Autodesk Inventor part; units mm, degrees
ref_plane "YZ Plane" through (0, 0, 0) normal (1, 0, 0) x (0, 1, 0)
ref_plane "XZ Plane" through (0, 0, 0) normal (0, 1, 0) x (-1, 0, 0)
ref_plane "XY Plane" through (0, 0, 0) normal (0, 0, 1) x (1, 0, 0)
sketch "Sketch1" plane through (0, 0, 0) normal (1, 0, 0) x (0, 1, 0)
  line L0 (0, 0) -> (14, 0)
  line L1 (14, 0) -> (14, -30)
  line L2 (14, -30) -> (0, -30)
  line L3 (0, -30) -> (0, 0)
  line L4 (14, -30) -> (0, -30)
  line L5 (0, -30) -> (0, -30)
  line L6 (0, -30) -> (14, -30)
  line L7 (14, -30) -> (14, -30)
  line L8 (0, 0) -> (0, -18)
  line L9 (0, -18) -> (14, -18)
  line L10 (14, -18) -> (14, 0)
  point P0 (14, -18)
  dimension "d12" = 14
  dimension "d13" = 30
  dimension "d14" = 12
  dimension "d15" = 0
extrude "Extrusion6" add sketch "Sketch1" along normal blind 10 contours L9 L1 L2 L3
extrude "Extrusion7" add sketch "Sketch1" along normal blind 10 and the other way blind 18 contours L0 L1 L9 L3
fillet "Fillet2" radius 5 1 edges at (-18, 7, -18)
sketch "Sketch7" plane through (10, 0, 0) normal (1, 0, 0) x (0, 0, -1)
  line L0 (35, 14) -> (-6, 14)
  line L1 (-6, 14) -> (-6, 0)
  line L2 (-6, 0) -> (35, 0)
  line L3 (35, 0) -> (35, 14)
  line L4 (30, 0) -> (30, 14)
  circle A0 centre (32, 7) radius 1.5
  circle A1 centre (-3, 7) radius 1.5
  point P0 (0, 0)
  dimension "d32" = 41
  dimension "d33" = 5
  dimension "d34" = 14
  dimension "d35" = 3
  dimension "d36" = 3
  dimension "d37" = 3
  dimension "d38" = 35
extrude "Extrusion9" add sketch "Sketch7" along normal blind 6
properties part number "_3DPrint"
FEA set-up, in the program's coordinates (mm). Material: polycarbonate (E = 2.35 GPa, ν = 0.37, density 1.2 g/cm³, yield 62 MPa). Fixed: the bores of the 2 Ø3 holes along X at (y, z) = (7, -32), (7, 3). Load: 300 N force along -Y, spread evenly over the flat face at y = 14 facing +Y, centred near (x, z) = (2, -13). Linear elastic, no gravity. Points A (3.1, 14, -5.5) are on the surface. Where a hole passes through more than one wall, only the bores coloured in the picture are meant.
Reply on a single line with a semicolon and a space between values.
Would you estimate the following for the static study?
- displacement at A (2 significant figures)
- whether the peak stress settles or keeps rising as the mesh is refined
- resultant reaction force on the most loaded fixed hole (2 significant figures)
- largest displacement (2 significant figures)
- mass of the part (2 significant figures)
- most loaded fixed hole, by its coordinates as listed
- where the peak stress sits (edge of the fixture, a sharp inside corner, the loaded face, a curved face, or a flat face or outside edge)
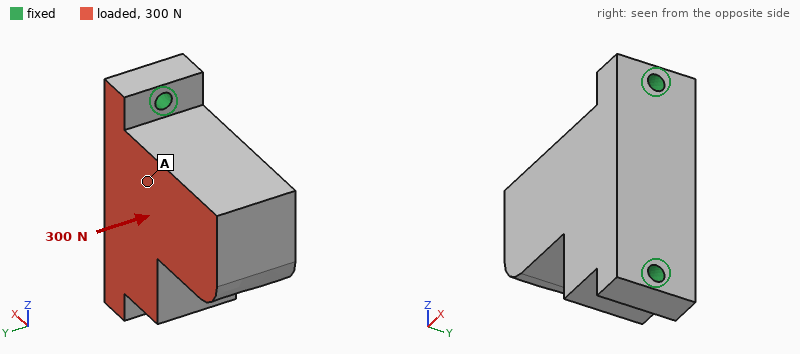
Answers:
0.20 mm; keeps rising; 170 N; 0.51 mm; 14 g; (7, 3); edge of the fixture
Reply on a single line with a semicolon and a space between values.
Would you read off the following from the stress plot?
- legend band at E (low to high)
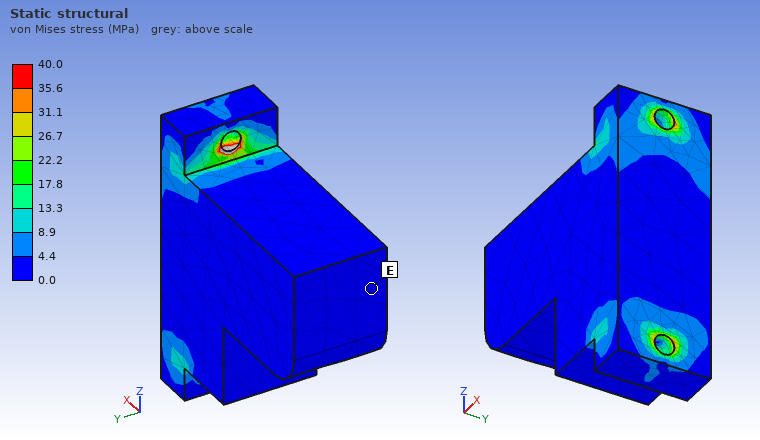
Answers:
0.0 to 4.4 MPa
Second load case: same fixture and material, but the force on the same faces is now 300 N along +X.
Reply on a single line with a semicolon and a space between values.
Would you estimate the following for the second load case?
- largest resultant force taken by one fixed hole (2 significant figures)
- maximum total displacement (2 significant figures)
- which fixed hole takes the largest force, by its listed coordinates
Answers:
180 N; 0.30 mm; (7, 3)
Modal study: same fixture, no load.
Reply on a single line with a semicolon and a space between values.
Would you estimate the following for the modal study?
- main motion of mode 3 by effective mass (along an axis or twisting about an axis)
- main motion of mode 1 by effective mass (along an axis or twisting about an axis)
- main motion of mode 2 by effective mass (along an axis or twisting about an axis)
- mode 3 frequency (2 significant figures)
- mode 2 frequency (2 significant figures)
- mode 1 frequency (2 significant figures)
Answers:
along X; along Y; along Z; 4700 Hz; 3700 Hz; 1300 Hz
